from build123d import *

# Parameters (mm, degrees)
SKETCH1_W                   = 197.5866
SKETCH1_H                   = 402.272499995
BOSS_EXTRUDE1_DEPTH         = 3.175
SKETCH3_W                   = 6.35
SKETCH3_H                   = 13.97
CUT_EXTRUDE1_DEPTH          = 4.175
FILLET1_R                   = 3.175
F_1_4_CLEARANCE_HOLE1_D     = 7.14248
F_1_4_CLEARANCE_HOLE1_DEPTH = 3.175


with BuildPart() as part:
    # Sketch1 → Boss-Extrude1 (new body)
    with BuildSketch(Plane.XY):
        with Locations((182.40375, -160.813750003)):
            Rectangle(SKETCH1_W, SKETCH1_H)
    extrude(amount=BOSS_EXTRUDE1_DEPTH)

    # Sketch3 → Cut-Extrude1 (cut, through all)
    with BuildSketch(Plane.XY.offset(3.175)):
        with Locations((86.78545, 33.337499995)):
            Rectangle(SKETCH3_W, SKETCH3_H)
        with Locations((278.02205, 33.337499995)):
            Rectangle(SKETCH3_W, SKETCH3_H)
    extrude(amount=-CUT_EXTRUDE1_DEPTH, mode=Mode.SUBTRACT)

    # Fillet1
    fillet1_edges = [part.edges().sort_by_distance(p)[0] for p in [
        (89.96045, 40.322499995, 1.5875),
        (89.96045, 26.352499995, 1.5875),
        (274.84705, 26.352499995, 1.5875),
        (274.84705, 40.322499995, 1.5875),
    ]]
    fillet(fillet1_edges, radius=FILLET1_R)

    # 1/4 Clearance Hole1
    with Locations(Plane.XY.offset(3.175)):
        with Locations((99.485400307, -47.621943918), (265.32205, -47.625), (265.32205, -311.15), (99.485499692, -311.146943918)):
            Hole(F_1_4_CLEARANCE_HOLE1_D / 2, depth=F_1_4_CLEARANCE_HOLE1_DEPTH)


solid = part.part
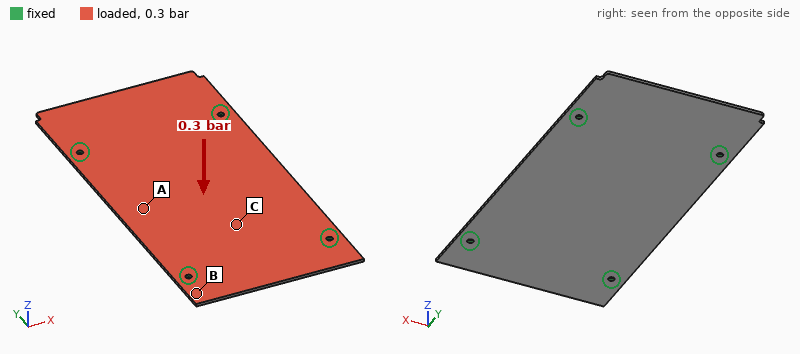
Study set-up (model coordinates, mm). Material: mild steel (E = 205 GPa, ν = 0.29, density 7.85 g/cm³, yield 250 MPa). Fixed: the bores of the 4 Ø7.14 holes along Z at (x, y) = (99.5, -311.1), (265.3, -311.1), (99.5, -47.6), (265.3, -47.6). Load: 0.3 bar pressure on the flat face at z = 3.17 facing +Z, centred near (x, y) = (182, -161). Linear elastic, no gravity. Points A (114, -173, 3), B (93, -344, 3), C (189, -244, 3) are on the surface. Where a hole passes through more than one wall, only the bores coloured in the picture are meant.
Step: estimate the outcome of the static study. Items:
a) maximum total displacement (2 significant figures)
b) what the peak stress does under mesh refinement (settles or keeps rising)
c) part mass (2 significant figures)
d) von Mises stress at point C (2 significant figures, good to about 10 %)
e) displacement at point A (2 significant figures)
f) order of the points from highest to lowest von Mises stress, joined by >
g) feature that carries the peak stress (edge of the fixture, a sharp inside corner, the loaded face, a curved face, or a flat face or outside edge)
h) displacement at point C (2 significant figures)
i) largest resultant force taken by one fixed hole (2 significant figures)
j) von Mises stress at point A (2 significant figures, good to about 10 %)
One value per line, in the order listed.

0.92 mm
keeps rising
2.0 kg
28 MPa
0.86 mm
A > C > B
edge of the fixture
0.67 mm
650 N
54 MPa
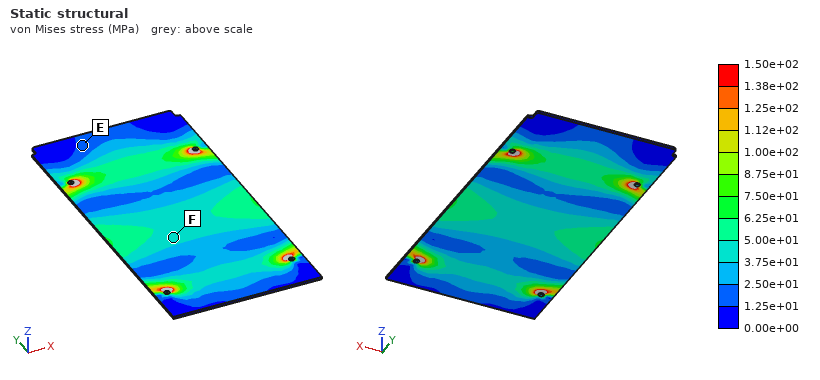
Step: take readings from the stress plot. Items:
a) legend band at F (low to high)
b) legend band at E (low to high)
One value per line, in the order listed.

3.75e+01 to 5.00e+01 MPa
1.25e+01 to 2.50e+01 MPa
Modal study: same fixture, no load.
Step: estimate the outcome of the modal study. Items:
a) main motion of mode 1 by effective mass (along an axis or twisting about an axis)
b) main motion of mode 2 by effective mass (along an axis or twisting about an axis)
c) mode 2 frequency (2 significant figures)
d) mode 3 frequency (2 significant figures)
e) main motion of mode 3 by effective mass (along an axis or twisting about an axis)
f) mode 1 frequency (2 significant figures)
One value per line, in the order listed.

along Z
along Z
270 Hz
320 Hz
twisting about Y
200 Hz
